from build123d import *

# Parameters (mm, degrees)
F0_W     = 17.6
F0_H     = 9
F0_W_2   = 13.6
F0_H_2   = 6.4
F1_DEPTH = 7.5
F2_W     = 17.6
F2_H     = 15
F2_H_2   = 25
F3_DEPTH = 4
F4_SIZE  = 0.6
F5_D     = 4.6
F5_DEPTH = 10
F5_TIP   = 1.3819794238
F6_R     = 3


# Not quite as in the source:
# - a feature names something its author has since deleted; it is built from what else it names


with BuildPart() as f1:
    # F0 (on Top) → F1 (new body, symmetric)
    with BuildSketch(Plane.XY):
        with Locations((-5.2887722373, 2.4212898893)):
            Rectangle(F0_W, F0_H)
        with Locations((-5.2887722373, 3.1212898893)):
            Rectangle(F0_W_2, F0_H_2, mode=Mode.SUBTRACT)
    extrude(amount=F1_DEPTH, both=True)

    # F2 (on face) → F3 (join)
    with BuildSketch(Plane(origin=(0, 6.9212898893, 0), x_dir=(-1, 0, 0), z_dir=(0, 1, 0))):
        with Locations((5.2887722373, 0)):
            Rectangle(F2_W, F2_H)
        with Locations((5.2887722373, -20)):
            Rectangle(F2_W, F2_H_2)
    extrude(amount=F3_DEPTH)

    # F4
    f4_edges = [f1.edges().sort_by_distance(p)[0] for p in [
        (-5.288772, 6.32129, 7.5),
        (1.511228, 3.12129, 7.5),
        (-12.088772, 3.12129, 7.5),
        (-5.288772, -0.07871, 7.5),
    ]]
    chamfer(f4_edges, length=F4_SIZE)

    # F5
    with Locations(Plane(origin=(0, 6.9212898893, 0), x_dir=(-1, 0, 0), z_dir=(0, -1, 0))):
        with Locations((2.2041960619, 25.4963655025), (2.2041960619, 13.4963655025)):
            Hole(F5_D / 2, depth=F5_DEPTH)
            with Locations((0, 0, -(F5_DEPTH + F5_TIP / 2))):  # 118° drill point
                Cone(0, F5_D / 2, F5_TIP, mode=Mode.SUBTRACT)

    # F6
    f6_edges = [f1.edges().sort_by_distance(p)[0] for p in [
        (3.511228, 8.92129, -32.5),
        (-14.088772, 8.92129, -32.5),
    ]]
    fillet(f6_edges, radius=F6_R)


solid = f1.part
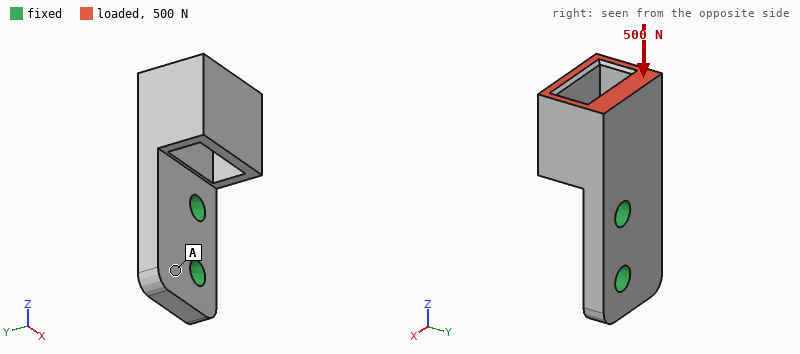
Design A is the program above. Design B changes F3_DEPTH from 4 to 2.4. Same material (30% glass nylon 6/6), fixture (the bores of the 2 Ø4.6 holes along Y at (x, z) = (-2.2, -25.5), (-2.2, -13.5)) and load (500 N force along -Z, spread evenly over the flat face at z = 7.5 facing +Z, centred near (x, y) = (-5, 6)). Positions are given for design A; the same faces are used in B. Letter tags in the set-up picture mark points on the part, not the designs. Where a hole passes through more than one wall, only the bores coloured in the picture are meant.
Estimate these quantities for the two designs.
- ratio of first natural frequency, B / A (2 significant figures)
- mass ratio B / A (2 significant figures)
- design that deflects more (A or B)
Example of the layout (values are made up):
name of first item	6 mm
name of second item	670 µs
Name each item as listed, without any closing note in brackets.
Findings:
ratio of first natural frequency, B / A	0.56
mass ratio B / A	0.71
design that deflects more	B
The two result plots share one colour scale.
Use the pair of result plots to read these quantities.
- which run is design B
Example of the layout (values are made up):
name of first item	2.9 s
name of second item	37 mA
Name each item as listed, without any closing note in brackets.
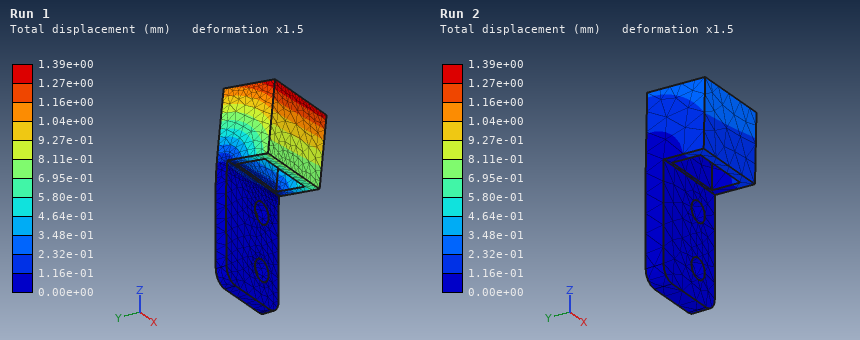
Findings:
which run is design B	Run 1
